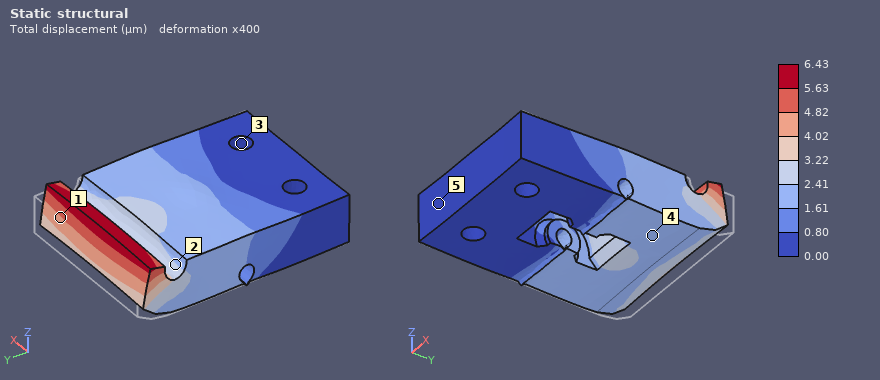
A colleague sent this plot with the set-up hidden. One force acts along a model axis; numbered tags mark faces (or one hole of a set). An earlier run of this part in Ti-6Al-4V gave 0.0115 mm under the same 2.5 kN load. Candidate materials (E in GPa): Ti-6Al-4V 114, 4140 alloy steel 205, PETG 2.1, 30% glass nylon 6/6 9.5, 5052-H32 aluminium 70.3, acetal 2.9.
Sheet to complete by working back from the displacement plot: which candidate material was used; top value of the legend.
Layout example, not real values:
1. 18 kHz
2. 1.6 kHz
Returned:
1. 4140 alloy steel
2. 6.43 µm
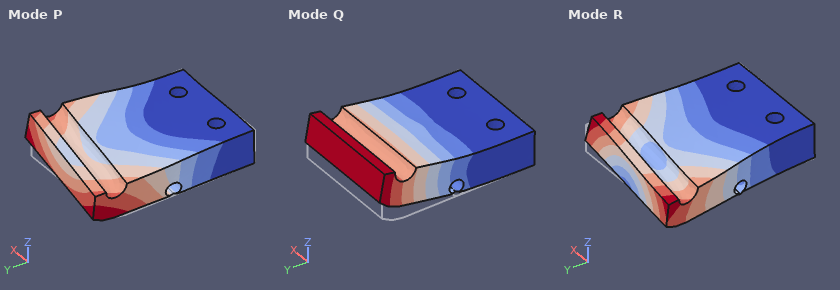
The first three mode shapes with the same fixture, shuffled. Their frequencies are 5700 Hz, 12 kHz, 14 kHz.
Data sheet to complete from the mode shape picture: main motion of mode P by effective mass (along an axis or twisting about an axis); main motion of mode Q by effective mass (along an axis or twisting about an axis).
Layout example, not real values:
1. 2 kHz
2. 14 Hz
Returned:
1. along X
2. along Z
